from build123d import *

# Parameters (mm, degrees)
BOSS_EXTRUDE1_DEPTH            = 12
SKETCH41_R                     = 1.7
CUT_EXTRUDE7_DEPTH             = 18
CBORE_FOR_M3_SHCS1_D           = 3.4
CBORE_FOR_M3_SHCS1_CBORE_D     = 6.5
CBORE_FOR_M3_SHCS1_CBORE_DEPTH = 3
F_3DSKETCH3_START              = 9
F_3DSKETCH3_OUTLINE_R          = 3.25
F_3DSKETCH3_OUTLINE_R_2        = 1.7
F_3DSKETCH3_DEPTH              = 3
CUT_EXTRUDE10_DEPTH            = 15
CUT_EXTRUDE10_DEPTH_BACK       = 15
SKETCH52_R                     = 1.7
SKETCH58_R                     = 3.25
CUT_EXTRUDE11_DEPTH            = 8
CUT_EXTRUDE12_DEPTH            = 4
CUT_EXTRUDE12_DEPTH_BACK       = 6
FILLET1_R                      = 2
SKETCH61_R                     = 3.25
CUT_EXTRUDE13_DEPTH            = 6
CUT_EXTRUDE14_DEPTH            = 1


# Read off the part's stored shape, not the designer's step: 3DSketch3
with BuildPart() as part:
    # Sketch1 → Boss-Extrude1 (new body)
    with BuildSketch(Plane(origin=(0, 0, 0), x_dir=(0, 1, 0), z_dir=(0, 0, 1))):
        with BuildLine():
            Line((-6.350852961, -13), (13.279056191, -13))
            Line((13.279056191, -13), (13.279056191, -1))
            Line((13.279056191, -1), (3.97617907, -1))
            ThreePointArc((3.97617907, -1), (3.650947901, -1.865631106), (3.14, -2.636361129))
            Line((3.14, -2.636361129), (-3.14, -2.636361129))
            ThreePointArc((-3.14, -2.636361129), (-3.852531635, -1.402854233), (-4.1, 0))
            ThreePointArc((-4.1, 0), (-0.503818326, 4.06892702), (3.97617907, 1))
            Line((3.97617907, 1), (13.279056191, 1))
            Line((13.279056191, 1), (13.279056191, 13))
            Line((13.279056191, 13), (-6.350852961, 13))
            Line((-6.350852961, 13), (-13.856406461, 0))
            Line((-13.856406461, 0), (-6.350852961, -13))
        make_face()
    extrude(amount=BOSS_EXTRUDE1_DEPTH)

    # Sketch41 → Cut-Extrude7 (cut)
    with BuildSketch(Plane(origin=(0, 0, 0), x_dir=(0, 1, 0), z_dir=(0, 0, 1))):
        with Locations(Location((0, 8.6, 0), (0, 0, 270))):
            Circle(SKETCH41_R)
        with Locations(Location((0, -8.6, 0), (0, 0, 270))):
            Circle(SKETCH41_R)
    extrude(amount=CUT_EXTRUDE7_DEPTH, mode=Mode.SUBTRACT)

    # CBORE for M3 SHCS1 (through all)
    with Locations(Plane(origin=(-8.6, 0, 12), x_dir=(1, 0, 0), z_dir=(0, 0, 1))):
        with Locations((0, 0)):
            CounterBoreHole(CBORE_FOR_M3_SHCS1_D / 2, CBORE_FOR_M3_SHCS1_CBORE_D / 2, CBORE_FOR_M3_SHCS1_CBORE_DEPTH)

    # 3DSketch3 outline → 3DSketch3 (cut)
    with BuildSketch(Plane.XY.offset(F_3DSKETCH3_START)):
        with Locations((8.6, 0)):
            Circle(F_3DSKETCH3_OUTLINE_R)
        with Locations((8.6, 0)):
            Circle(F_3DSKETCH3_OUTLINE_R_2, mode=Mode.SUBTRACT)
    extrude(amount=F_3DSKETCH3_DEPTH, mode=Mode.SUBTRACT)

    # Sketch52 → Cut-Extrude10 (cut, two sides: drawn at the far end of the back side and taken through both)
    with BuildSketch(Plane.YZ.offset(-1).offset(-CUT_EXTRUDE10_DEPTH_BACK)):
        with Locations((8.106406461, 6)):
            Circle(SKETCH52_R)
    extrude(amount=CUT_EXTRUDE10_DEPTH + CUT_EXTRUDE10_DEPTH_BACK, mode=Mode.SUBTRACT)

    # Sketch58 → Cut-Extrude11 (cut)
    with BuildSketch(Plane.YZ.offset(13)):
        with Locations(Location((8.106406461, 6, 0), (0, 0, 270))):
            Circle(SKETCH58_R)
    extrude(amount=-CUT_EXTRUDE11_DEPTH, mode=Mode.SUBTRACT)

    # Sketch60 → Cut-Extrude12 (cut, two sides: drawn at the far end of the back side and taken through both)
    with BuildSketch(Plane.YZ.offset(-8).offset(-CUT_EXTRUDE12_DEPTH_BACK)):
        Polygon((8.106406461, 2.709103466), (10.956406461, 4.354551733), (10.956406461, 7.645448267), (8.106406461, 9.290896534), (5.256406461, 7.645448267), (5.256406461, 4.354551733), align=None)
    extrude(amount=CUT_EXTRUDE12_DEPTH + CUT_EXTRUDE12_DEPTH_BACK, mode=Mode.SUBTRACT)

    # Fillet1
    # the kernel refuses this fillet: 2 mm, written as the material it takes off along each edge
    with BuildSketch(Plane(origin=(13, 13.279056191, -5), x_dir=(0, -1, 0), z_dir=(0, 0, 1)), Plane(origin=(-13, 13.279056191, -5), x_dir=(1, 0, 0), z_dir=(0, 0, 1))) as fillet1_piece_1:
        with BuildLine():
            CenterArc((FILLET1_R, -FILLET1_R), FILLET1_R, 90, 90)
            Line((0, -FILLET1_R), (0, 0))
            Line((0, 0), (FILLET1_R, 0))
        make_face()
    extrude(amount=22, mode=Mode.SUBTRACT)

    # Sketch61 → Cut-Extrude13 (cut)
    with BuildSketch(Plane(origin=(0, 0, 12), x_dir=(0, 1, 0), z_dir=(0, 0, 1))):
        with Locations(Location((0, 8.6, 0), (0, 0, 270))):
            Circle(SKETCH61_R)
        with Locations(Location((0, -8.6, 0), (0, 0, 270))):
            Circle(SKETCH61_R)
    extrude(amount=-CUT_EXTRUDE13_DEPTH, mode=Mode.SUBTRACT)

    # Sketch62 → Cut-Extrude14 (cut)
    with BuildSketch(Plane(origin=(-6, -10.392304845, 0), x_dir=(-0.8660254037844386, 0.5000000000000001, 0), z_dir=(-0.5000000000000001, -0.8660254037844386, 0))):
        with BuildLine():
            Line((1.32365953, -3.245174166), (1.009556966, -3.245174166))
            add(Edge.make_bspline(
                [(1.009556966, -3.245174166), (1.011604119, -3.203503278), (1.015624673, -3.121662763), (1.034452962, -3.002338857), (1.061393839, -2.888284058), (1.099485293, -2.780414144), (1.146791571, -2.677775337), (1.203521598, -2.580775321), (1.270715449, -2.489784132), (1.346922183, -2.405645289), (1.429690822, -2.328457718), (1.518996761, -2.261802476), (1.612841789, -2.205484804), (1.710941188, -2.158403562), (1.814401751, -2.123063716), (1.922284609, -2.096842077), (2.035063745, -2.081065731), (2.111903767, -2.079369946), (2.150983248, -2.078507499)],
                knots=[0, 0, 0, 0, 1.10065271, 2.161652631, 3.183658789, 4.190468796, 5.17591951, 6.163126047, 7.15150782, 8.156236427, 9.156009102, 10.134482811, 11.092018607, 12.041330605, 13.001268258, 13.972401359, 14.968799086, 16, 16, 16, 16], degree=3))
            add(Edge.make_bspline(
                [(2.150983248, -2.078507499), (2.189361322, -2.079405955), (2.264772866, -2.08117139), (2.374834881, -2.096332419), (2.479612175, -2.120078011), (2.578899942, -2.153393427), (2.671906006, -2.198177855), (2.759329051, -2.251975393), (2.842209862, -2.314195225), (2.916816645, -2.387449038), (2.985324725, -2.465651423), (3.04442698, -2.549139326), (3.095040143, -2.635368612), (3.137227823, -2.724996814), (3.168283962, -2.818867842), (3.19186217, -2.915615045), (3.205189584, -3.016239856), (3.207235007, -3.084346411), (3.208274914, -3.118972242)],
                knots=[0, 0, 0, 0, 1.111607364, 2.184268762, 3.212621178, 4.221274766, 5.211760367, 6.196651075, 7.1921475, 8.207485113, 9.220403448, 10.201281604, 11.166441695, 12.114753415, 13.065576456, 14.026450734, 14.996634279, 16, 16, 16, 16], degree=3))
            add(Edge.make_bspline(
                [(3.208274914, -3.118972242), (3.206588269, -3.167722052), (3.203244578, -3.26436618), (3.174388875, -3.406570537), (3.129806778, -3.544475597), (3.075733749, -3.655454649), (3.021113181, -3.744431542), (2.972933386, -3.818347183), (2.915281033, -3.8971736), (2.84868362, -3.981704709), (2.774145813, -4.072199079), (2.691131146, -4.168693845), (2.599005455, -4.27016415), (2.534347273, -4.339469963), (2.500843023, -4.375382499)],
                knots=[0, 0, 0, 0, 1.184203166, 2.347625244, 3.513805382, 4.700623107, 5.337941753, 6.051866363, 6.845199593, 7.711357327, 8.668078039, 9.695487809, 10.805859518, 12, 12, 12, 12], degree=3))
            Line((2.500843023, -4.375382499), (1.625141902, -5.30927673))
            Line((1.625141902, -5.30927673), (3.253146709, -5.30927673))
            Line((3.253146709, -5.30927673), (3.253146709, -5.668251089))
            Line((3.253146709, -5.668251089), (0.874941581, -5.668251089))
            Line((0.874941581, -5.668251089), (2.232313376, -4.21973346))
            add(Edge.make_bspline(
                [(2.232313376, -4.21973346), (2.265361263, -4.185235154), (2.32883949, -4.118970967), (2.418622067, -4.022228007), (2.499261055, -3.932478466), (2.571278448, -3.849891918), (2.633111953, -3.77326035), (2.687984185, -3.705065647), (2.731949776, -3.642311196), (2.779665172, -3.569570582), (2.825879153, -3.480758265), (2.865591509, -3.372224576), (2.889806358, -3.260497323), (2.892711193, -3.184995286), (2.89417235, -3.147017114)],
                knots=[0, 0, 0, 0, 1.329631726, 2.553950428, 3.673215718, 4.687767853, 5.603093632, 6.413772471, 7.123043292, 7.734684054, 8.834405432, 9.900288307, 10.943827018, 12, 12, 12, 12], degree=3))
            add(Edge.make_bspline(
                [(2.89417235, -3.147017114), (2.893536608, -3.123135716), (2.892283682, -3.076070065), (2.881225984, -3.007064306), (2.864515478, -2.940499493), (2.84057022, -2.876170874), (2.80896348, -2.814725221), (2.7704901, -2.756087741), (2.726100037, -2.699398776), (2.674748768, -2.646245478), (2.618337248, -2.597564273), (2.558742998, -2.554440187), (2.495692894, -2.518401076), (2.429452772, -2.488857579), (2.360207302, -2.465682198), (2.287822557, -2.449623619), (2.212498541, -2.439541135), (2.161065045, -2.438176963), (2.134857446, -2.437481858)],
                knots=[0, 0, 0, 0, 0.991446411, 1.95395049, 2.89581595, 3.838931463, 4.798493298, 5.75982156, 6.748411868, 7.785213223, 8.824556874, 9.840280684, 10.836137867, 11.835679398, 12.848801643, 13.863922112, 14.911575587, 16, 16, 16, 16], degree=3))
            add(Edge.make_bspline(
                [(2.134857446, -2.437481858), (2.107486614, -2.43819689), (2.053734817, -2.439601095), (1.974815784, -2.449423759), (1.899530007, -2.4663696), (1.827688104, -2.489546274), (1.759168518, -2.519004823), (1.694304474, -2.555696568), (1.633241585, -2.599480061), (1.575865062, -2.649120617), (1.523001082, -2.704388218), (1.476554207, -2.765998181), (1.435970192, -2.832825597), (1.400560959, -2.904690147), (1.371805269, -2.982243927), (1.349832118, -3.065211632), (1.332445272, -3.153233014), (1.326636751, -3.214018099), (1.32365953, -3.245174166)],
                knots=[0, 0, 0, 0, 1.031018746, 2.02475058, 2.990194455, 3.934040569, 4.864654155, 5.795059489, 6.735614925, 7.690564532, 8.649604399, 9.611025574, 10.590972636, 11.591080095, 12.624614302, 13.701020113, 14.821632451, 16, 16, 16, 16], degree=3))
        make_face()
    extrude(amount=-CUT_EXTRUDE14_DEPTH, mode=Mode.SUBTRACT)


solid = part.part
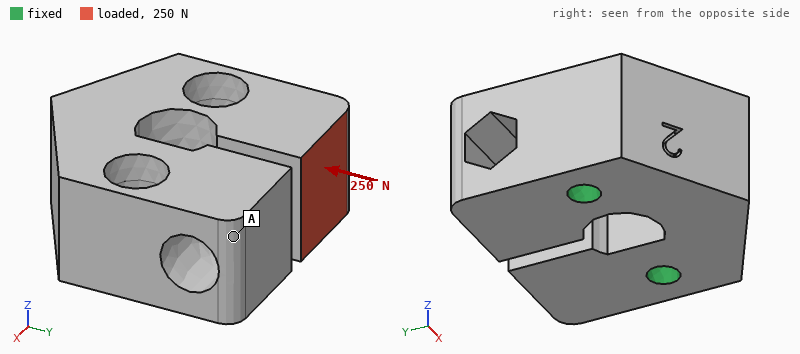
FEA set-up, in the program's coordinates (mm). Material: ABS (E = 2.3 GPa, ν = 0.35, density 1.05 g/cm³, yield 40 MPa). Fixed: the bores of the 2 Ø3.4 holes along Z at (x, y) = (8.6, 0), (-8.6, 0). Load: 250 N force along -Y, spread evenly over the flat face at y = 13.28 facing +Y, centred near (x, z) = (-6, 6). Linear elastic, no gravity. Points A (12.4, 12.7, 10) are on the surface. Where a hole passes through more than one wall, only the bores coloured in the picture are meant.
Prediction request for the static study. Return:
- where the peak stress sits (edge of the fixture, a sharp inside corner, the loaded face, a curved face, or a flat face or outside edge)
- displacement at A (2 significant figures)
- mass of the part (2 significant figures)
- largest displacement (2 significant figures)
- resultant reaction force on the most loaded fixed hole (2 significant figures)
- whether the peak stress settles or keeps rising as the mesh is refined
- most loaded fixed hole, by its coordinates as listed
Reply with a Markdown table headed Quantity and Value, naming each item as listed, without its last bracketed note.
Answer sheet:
| Quantity | Value |
|---|---|
| where the peak stress sits | edge of the fixture |
| displacement at A | 14 µm |
| mass of the part | 5.7 g |
| largest displacement | 93 µm |
| resultant reaction force on the most loaded fixed hole | 230 N |
| whether the peak stress settles or keeps rising as the mesh is refined | keeps rising |
| most loaded fixed hole, by its coordinates as listed | (-8.6, 0) |
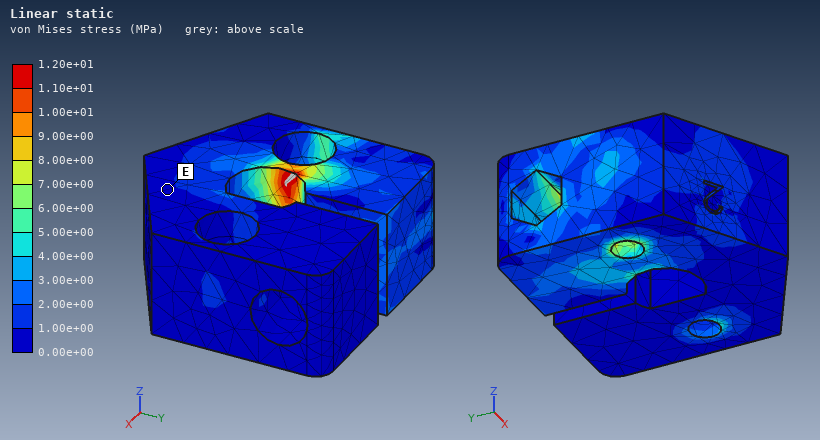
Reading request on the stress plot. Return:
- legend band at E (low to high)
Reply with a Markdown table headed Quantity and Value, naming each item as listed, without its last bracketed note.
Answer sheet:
| Quantity | Value |
|---|---|
| legend band at E | 0.00e+00 to 1.00e+00 MPa |
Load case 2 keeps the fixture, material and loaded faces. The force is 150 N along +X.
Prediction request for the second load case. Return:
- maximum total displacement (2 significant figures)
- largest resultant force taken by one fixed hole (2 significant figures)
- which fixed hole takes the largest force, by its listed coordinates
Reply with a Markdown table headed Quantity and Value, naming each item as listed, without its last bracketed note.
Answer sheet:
| Quantity | Value |
|---|---|
| maximum total displacement | 0.22 mm |
| largest resultant force taken by one fixed hole | 210 N |
| which fixed hole takes the largest force, by its listed coordinates | (-8.6, 0) |
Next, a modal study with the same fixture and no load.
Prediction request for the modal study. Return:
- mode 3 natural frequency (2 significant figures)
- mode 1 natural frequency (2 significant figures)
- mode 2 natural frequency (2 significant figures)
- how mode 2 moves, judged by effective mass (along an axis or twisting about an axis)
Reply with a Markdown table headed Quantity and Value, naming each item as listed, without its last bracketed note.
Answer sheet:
| Quantity | Value |
|---|---|
| mode 3 natural frequency | 6000 Hz |
| mode 1 natural frequency | 5000 Hz |
| mode 2 natural frequency | 5700 Hz |
| how mode 2 moves, judged by effective mass | along X |
